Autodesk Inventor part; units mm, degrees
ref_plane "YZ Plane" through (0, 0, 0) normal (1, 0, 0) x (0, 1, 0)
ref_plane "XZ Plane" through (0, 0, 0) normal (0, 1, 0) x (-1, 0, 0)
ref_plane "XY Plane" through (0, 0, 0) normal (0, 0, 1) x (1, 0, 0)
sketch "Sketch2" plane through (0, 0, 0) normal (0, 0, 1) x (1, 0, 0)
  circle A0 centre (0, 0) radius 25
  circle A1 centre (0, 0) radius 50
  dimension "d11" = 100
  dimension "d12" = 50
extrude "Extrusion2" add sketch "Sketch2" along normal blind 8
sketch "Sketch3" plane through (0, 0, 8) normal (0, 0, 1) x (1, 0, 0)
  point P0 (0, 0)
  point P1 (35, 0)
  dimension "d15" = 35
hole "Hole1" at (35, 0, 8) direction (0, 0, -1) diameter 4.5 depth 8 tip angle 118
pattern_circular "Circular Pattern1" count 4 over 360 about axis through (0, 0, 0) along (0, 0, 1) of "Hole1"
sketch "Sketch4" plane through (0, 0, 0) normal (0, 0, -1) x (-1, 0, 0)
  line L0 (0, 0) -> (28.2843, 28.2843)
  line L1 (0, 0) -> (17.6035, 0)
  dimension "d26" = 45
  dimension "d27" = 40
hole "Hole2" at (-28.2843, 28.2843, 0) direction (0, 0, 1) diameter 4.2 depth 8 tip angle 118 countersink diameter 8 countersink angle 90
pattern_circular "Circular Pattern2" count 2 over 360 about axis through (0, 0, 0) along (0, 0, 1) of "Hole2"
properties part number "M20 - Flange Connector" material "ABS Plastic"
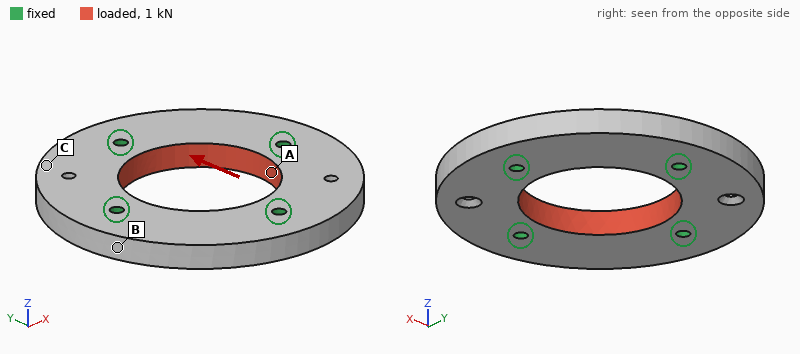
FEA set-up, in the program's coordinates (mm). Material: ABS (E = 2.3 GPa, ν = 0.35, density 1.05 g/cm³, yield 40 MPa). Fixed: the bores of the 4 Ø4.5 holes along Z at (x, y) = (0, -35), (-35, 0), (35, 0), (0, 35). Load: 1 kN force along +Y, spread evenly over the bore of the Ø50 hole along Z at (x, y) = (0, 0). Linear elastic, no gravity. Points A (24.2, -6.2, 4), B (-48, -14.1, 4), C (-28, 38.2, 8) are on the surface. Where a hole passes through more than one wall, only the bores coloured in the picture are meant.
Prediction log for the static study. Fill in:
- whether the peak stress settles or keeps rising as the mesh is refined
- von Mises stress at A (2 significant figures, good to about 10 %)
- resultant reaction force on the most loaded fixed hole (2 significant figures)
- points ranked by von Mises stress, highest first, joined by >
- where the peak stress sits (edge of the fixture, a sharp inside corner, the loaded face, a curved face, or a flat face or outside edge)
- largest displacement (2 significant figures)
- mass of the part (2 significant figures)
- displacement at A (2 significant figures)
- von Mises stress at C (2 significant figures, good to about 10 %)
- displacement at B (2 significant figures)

keeps rising
1.4 MPa
270 N
A > C > B
edge of the fixture
17 µm
49 g
15 µm
0.60 MPa
3.2 µm
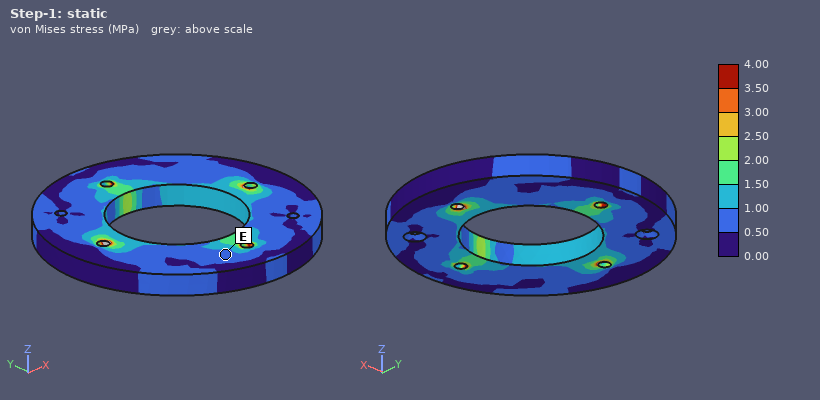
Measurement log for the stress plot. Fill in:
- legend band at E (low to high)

0.50 to 1.00 MPa
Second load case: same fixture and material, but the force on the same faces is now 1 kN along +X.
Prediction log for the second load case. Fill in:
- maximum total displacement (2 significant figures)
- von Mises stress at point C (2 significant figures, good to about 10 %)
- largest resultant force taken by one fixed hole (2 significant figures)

17 µm
0.59 MPa
270 N
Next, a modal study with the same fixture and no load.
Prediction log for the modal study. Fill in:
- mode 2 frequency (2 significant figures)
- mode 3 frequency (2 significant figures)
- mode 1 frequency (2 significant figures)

2300 Hz
2400 Hz
2100 Hz
